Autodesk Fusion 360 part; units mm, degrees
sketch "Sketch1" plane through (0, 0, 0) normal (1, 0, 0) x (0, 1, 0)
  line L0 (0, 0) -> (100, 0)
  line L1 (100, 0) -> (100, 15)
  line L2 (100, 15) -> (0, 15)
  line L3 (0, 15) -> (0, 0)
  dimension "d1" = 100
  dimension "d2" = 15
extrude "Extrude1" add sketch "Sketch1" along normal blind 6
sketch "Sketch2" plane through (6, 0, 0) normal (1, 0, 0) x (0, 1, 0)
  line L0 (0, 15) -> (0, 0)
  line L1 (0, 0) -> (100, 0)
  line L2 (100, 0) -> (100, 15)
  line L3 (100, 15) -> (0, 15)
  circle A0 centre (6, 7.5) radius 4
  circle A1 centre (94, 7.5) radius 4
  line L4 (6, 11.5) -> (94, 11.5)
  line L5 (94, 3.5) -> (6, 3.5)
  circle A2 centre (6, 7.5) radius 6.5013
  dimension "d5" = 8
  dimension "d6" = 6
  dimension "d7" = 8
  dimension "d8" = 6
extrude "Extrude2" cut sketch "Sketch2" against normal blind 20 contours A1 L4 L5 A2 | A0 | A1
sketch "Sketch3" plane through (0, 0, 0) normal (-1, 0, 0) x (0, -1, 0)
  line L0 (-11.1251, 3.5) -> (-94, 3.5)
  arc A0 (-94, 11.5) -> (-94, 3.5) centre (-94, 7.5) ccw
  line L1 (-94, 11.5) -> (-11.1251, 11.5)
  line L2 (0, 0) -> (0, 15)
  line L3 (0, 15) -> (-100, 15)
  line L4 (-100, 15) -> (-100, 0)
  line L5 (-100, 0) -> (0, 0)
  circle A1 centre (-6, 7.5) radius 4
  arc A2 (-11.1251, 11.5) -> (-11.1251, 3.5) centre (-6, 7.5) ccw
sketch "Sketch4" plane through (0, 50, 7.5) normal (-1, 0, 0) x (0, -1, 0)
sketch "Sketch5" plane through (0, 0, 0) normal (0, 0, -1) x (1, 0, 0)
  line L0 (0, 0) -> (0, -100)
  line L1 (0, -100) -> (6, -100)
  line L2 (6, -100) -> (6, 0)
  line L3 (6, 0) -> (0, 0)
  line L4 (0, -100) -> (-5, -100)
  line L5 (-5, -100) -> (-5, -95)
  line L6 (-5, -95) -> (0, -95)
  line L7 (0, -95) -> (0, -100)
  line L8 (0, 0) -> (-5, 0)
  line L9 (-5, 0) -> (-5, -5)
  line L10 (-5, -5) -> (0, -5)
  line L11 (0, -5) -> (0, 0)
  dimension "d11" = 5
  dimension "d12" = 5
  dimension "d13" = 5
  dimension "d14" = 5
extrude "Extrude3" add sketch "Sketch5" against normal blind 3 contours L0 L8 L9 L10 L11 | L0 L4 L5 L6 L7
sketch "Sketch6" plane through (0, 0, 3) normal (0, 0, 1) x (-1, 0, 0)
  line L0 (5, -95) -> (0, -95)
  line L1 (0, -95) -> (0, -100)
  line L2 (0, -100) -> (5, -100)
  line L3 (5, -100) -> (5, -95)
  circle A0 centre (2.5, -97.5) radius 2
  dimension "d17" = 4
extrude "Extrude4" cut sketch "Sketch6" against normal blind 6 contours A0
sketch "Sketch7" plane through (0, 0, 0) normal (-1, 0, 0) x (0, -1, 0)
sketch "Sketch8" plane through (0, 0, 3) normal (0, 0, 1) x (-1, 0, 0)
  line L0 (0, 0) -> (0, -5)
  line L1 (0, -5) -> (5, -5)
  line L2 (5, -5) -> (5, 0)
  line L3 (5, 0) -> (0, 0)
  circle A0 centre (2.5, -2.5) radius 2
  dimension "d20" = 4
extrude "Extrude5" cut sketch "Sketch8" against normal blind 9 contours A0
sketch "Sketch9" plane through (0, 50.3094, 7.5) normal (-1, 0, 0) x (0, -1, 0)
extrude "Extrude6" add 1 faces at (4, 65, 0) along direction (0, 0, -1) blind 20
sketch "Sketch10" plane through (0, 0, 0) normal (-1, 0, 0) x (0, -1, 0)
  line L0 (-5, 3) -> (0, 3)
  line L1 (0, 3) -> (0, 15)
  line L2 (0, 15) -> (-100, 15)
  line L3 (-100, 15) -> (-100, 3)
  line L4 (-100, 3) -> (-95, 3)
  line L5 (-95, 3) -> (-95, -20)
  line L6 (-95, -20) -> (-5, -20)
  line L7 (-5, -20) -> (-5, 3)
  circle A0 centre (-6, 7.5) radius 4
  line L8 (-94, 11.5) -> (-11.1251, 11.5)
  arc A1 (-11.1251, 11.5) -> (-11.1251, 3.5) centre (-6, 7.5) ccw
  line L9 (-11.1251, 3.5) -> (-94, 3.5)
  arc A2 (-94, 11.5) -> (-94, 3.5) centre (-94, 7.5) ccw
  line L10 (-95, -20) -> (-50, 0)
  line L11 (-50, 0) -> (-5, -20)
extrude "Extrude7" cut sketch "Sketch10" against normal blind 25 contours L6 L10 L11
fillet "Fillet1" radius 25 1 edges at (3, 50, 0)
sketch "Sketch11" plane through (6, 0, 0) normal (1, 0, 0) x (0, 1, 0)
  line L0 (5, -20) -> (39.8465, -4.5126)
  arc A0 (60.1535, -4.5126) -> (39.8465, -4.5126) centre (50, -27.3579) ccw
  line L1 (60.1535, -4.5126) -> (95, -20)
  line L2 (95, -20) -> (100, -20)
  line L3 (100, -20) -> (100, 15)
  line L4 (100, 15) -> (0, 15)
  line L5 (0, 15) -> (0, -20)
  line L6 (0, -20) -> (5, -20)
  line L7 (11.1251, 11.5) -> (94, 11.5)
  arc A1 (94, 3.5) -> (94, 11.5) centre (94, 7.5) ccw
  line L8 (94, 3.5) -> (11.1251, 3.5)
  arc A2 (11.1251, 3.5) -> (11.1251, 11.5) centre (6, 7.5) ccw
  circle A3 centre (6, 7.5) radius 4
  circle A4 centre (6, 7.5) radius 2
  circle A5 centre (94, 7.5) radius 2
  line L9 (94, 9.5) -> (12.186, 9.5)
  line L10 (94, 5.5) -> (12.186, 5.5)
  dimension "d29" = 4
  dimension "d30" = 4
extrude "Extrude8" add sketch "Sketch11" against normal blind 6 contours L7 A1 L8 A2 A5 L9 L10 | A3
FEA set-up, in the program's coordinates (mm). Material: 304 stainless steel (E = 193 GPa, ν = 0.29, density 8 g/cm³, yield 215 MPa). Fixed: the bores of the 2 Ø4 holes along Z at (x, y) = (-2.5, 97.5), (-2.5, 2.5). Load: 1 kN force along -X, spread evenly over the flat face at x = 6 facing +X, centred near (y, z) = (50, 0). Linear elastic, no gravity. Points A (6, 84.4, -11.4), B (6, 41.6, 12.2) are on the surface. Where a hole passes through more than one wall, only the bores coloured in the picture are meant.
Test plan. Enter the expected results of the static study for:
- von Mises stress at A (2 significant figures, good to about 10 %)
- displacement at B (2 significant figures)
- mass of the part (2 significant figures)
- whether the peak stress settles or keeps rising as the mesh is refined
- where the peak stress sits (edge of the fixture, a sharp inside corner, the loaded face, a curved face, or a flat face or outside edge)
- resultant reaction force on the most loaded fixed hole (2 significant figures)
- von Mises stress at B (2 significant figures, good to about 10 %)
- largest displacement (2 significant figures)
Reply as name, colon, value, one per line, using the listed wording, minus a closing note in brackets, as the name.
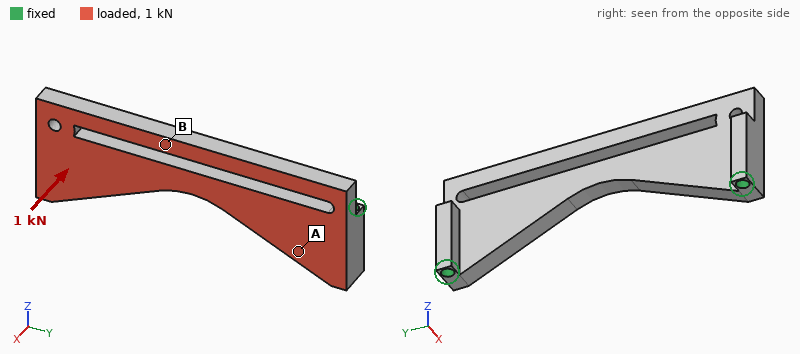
von Mises stress at A: 15 MPa
displacement at B: 49 µm
mass of the part: 110 g
whether the peak stress settles or keeps rising as the mesh is refined: keeps rising
where the peak stress sits: a sharp inside corner
resultant reaction force on the most loaded fixed hole: 630 N
von Mises stress at B: 35 MPa
largest displacement: 55 µm
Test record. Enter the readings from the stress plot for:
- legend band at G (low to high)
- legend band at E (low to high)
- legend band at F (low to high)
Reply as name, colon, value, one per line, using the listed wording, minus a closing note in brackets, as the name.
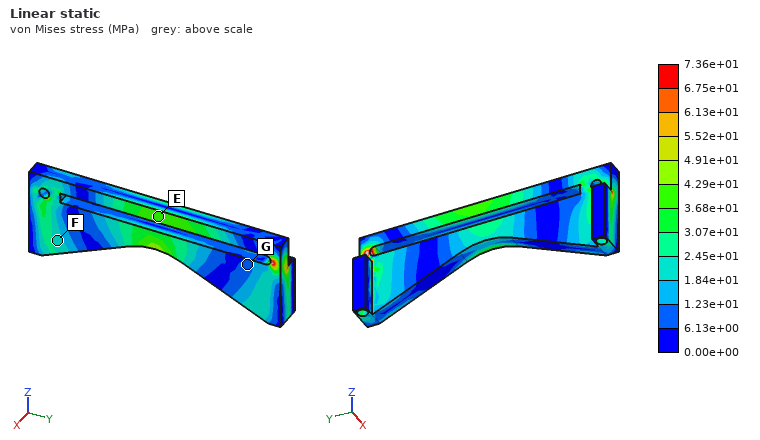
legend band at G: 6.13e+00 to 1.23e+01 MPa
legend band at E: 3.68e+01 to 4.29e+01 MPa
legend band at F: 1.84e+01 to 2.45e+01 MPa
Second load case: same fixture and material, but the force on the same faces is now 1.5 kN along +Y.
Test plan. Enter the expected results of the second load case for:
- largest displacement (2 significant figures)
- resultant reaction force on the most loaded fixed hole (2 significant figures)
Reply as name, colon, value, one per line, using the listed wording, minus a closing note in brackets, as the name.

largest displacement: 5.6 µm
resultant reaction force on the most loaded fixed hole: 780 N
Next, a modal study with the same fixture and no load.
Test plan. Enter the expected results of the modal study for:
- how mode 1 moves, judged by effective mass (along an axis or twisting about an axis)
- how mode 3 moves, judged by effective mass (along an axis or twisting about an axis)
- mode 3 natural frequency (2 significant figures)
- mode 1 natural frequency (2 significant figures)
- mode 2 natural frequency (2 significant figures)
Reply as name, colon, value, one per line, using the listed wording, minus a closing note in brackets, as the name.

how mode 1 moves, judged by effective mass: along X
how mode 3 moves, judged by effective mass: along X
mode 3 natural frequency: 3600 Hz
mode 1 natural frequency: 2600 Hz
mode 2 natural frequency: 3100 Hz
